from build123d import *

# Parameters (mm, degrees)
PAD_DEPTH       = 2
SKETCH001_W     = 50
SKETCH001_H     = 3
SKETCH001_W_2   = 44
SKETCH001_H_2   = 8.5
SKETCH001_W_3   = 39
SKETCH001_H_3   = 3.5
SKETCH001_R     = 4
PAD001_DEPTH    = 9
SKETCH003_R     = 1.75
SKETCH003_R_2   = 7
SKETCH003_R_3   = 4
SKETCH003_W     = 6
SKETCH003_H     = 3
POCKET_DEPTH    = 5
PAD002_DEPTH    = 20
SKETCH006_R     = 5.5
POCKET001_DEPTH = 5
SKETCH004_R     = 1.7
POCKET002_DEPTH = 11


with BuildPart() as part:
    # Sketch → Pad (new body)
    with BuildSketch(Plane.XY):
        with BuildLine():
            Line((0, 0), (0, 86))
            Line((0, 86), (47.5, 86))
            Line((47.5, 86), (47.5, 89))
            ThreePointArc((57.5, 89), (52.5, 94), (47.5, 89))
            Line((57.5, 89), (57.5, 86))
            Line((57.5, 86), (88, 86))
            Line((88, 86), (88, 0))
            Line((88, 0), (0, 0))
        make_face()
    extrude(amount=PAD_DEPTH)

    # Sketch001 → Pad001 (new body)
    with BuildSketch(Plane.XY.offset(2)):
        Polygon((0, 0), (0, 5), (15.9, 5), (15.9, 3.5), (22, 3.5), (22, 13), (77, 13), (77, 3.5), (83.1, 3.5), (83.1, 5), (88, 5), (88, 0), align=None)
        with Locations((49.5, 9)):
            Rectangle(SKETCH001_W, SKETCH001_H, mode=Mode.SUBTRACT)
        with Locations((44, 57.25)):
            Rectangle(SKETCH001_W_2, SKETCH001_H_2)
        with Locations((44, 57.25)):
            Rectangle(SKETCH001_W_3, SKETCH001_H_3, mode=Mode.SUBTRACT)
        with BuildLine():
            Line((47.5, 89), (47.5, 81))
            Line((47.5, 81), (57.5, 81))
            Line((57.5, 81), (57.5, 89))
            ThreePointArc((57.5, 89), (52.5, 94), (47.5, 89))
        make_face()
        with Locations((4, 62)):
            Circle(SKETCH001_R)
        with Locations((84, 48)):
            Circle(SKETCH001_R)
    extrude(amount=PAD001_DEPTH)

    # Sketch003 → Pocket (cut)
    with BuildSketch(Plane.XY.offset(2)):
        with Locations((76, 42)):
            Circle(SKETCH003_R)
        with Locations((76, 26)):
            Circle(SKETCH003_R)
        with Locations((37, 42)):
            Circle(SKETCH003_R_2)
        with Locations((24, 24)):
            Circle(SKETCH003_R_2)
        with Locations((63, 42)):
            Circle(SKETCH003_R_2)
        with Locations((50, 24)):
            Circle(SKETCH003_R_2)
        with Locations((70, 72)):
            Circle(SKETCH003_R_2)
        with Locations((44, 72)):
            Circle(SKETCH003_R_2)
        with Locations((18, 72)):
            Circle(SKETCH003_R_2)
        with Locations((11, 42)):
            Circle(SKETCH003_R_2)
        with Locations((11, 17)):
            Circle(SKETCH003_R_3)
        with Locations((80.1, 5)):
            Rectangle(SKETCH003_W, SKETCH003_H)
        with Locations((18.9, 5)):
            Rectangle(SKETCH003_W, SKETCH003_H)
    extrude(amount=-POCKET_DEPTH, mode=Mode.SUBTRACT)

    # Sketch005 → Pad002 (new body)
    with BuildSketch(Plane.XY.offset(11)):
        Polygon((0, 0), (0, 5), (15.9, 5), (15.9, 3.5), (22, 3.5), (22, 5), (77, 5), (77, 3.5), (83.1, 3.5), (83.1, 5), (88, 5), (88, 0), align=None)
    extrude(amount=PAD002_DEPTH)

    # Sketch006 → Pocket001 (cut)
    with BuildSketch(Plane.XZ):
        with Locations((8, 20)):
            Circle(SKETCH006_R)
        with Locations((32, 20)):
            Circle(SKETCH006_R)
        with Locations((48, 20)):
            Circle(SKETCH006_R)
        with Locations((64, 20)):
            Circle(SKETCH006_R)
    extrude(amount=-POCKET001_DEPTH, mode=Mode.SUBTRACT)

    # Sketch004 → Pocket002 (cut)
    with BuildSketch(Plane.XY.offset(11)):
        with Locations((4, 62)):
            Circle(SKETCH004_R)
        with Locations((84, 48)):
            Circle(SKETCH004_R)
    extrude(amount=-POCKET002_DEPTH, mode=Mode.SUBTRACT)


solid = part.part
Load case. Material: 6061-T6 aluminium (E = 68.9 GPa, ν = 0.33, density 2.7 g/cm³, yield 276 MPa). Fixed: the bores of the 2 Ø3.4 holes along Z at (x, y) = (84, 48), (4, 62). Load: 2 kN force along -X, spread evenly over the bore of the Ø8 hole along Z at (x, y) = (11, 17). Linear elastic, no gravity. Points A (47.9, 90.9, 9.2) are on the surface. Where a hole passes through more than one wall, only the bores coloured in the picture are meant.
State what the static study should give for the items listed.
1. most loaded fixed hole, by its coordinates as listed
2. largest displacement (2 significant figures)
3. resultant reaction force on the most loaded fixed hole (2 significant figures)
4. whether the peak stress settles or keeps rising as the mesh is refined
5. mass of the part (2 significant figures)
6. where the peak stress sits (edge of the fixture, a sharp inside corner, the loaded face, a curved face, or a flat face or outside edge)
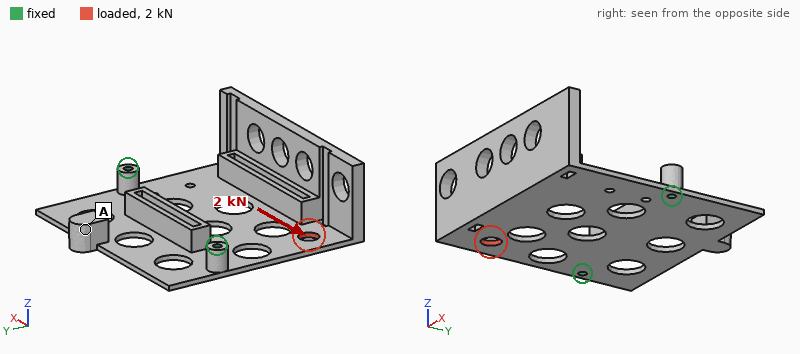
(84, 48)
70 µm
1.4 kN
keeps rising
80 g
edge of the fixture
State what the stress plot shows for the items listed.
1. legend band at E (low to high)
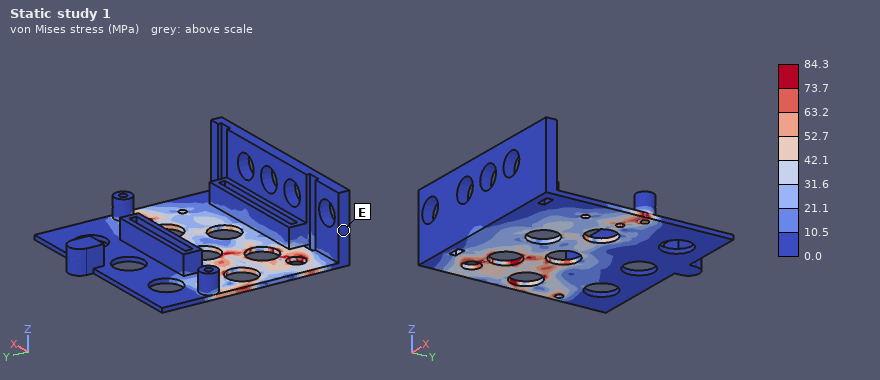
0.0 to 10.5 MPa
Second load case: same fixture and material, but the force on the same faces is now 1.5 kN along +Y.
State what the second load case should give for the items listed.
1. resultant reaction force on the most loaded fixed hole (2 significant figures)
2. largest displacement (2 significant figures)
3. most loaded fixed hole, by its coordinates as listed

1.4 kN
54 µm
(4, 62)
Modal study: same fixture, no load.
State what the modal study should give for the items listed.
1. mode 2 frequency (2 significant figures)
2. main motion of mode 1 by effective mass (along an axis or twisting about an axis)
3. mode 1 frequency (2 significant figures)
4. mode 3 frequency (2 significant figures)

510 Hz
along Z
170 Hz
780 Hz
